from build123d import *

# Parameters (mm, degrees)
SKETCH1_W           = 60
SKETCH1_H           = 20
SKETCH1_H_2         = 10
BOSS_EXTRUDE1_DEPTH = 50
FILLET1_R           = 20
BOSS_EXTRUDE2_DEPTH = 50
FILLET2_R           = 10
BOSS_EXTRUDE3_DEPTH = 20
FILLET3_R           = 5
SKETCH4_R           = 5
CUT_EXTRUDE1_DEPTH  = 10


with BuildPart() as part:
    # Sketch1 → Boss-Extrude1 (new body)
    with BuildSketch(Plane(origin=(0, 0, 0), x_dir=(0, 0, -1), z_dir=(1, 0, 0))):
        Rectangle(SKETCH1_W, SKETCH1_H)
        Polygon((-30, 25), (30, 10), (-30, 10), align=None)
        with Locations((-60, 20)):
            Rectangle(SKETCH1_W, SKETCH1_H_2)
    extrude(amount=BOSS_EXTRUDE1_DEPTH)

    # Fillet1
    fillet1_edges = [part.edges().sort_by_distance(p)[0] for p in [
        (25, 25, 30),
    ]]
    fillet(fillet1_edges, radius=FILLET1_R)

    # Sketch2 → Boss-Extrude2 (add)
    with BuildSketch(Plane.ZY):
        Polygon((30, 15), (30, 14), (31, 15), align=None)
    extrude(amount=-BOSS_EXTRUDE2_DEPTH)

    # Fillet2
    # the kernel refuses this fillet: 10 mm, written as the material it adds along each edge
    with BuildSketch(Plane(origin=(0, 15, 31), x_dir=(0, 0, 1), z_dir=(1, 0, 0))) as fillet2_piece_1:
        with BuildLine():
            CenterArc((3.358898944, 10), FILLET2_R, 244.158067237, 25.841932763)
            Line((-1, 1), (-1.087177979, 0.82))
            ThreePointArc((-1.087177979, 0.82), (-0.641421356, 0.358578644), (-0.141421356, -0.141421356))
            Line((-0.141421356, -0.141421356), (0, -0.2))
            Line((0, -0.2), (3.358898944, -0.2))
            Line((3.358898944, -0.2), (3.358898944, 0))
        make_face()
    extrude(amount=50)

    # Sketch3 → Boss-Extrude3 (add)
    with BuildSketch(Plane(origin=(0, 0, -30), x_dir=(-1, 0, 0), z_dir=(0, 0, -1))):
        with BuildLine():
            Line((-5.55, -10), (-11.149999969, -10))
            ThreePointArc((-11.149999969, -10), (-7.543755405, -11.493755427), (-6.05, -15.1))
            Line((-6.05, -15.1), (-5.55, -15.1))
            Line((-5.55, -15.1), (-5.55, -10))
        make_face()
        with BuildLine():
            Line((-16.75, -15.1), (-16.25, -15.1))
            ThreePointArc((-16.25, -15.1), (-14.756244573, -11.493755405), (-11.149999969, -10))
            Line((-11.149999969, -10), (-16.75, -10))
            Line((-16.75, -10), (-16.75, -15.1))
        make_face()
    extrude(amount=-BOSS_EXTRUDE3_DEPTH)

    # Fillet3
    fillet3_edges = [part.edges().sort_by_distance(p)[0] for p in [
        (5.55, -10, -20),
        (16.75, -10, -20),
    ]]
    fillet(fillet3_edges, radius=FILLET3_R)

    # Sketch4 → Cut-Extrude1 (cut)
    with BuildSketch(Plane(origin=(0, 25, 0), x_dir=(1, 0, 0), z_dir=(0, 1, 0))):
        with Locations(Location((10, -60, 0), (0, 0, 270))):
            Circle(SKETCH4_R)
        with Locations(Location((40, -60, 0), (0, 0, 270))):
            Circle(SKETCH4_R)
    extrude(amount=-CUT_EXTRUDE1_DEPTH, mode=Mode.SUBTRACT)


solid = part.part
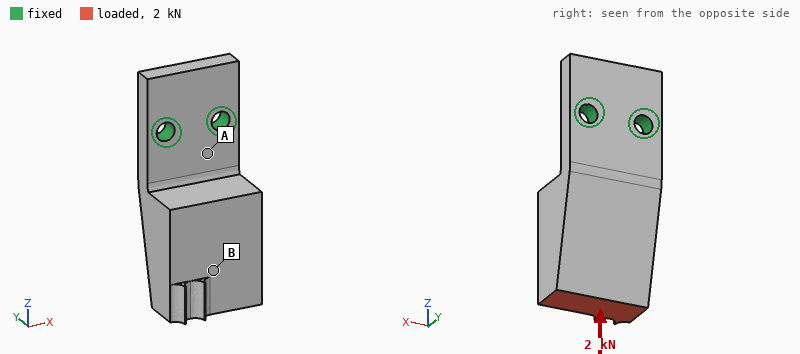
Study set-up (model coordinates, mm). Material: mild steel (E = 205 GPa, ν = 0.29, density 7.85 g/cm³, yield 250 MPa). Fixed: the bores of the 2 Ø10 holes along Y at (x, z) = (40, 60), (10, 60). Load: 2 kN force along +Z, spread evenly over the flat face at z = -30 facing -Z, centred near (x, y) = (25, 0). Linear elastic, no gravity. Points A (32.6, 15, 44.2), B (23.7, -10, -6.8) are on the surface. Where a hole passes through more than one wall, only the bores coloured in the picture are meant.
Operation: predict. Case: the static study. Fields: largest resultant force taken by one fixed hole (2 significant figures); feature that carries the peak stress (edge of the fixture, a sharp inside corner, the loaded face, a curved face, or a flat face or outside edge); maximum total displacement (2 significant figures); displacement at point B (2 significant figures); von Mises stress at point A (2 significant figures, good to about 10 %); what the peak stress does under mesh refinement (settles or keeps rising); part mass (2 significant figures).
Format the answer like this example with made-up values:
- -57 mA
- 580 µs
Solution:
- 1.0 kN
- edge of the fixture
- 0.12 mm
- 0.085 mm
- 48 MPa
- keeps rising
- 880 g
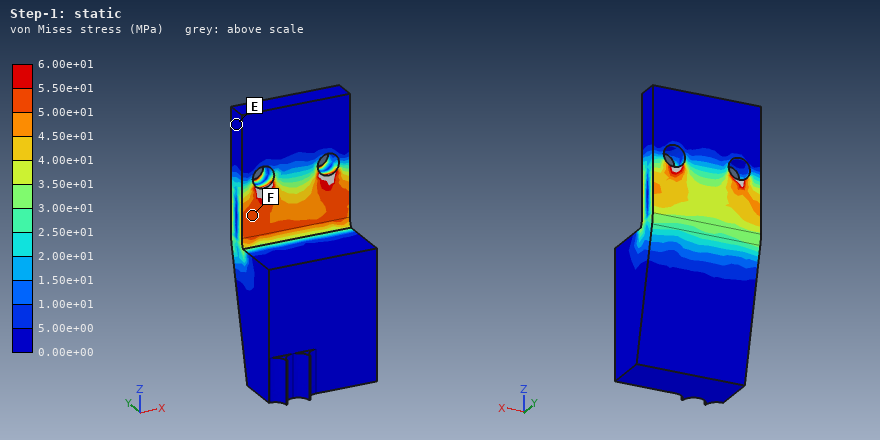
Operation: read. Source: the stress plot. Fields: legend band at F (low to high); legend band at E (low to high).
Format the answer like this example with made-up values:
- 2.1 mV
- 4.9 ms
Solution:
- 5.00e+01 to 5.50e+01 MPa
- 0.00e+00 to 5.00e+00 MPa
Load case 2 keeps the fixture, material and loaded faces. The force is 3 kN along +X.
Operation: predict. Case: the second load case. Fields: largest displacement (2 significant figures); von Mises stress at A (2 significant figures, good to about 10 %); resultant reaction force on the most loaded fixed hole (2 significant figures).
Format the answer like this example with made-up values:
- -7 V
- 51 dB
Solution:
- 56 µm
- 49 MPa
- 8.0 kN
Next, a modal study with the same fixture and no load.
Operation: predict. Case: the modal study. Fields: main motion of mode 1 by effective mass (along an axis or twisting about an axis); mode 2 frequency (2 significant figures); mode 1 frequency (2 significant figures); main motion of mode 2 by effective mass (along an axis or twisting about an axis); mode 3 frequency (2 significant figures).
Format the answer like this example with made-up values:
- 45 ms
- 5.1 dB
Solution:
- along Y
- 2100 Hz
- 690 Hz
- along X
- 3900 Hz
